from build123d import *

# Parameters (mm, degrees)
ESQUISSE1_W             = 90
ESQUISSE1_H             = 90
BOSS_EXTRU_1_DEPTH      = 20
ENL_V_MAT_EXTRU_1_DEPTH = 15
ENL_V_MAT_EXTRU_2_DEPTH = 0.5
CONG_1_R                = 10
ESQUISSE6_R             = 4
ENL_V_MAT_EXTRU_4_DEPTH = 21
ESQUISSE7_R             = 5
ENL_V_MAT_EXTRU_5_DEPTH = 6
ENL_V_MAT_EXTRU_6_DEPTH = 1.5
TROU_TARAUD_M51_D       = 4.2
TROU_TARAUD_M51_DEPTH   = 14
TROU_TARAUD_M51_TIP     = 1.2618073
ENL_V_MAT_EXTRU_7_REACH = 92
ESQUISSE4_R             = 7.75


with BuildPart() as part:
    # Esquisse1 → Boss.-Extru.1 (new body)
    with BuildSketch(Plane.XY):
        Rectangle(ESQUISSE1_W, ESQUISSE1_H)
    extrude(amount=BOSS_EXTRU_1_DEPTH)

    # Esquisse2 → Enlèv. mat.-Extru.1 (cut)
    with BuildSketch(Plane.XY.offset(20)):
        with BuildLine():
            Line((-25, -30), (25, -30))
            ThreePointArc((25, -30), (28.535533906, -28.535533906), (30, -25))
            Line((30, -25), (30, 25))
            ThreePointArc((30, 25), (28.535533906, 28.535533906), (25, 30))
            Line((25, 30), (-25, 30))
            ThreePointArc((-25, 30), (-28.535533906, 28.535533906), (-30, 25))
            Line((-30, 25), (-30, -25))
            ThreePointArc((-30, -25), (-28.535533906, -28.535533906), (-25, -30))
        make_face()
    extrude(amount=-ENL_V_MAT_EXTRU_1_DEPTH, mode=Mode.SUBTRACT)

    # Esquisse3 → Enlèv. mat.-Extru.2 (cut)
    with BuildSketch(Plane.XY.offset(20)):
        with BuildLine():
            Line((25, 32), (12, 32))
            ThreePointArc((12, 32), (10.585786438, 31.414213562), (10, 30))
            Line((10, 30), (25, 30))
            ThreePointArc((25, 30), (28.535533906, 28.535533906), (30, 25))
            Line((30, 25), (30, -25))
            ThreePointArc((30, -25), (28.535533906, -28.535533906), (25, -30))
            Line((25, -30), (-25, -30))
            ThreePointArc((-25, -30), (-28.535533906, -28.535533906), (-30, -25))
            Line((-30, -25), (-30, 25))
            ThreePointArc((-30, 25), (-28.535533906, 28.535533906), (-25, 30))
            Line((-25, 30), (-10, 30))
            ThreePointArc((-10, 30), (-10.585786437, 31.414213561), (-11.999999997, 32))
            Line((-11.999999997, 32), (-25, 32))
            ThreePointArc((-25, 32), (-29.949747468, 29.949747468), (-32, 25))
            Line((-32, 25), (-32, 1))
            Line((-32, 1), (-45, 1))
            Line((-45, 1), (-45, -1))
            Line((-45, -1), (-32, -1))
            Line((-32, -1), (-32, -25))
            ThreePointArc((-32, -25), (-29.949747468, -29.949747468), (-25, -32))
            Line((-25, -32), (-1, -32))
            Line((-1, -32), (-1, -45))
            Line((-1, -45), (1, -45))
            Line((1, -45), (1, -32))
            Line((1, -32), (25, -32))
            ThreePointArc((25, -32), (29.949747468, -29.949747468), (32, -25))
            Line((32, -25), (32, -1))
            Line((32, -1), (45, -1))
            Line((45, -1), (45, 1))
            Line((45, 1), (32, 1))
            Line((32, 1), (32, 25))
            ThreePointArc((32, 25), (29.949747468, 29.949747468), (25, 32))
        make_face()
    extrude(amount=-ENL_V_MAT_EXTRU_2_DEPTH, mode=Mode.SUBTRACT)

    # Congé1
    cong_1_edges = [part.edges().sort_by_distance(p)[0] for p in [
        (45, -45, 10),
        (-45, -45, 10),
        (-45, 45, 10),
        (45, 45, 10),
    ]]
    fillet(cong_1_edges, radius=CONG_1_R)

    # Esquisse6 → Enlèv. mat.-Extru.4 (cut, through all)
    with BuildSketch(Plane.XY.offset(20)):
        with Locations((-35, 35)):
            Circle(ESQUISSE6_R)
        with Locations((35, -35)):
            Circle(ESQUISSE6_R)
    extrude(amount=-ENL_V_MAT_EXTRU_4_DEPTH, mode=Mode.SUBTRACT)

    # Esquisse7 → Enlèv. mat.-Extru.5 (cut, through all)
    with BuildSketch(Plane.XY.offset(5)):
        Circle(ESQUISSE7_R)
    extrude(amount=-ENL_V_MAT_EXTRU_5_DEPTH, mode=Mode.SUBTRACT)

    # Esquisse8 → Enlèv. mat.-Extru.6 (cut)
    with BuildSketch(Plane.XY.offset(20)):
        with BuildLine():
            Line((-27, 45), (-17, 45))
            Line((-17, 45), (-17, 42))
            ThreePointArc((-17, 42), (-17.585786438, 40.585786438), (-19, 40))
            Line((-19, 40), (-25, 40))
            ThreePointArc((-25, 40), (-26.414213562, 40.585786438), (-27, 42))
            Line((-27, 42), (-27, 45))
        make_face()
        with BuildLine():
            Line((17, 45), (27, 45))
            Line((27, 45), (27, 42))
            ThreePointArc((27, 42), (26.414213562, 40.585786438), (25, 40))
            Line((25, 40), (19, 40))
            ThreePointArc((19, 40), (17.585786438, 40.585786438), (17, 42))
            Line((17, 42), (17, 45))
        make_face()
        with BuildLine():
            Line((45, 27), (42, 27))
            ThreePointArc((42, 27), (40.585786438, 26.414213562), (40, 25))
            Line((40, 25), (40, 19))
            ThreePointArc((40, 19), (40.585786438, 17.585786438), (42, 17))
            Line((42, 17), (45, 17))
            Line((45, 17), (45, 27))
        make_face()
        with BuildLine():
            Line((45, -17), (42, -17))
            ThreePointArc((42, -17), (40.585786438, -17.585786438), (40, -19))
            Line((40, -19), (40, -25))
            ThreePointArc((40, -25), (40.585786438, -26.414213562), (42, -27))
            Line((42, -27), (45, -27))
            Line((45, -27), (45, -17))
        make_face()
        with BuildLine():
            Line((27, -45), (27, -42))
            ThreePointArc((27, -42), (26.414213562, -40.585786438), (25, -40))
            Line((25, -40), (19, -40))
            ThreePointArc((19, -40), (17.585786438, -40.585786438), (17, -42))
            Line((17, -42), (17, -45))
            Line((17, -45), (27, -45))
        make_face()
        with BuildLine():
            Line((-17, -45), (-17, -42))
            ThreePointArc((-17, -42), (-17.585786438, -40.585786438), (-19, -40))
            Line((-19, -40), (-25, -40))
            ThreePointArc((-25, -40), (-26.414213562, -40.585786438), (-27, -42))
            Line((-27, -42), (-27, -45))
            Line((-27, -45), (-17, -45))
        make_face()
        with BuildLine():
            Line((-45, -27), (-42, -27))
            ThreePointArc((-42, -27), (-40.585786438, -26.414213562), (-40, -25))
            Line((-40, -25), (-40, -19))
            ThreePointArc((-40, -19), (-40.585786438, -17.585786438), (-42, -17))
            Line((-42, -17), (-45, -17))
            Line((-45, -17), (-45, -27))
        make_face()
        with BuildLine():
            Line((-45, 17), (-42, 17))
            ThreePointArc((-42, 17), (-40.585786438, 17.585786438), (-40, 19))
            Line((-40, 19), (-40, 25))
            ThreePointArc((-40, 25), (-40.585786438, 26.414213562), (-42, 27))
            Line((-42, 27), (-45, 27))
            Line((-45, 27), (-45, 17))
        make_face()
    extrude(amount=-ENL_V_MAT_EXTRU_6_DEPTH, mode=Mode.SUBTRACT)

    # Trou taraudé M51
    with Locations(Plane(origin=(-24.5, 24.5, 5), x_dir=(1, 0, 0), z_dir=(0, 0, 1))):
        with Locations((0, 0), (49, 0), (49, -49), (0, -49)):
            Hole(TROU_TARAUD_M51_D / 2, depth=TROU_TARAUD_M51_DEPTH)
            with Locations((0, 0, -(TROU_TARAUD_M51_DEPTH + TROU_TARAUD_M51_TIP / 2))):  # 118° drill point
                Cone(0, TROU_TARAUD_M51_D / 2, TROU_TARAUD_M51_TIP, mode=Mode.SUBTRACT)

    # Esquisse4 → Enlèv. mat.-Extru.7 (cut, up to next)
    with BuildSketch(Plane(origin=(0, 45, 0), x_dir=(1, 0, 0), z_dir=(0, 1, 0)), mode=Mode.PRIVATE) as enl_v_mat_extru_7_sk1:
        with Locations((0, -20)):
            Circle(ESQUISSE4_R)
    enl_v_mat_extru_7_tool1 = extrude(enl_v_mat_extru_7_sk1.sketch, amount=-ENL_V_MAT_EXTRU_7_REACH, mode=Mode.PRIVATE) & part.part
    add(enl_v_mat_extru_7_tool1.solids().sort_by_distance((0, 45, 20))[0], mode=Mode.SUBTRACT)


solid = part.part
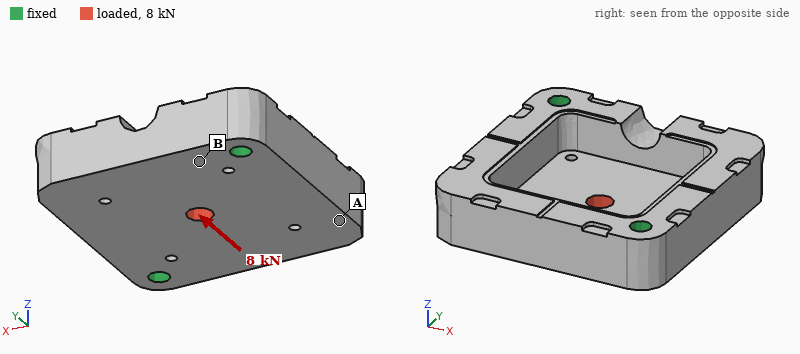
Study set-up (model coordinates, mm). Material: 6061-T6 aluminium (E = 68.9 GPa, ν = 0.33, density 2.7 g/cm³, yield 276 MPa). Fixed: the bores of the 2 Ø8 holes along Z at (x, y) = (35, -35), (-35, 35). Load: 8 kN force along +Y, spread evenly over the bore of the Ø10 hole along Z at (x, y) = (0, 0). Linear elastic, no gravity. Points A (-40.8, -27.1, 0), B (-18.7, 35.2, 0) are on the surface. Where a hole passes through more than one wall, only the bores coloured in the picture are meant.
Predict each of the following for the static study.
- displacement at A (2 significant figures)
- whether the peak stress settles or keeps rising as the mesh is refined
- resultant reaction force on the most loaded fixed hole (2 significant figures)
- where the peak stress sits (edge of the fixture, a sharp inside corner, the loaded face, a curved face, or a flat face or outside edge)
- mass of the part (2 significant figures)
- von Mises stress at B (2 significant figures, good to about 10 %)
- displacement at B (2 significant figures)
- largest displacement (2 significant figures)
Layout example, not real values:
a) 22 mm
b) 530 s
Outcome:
a) 23 µm
b) keeps rising
c) 4.0 kN
d) a sharp inside corner
e) 270 g
f) 22 MPa
g) 8.5 µm
h) 33 µm
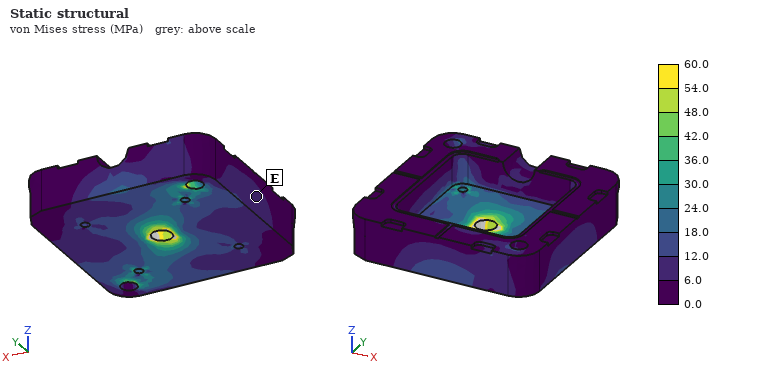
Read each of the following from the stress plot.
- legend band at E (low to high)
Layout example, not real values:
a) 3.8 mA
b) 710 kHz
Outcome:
a) 6.0 to 12.0 MPa
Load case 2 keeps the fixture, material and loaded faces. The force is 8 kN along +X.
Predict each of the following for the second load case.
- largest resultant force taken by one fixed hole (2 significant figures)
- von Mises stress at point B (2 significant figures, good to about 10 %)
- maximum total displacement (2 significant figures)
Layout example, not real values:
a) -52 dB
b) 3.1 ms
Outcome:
a) 4.0 kN
b) 16 MPa
c) 31 µm
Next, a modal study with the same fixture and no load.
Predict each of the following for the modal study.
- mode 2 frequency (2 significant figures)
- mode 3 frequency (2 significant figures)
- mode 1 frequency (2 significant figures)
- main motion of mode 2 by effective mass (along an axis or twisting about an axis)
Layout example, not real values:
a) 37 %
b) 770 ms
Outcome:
a) 3900 Hz
b) 7900 Hz
c) 3300 Hz
d) along Z
